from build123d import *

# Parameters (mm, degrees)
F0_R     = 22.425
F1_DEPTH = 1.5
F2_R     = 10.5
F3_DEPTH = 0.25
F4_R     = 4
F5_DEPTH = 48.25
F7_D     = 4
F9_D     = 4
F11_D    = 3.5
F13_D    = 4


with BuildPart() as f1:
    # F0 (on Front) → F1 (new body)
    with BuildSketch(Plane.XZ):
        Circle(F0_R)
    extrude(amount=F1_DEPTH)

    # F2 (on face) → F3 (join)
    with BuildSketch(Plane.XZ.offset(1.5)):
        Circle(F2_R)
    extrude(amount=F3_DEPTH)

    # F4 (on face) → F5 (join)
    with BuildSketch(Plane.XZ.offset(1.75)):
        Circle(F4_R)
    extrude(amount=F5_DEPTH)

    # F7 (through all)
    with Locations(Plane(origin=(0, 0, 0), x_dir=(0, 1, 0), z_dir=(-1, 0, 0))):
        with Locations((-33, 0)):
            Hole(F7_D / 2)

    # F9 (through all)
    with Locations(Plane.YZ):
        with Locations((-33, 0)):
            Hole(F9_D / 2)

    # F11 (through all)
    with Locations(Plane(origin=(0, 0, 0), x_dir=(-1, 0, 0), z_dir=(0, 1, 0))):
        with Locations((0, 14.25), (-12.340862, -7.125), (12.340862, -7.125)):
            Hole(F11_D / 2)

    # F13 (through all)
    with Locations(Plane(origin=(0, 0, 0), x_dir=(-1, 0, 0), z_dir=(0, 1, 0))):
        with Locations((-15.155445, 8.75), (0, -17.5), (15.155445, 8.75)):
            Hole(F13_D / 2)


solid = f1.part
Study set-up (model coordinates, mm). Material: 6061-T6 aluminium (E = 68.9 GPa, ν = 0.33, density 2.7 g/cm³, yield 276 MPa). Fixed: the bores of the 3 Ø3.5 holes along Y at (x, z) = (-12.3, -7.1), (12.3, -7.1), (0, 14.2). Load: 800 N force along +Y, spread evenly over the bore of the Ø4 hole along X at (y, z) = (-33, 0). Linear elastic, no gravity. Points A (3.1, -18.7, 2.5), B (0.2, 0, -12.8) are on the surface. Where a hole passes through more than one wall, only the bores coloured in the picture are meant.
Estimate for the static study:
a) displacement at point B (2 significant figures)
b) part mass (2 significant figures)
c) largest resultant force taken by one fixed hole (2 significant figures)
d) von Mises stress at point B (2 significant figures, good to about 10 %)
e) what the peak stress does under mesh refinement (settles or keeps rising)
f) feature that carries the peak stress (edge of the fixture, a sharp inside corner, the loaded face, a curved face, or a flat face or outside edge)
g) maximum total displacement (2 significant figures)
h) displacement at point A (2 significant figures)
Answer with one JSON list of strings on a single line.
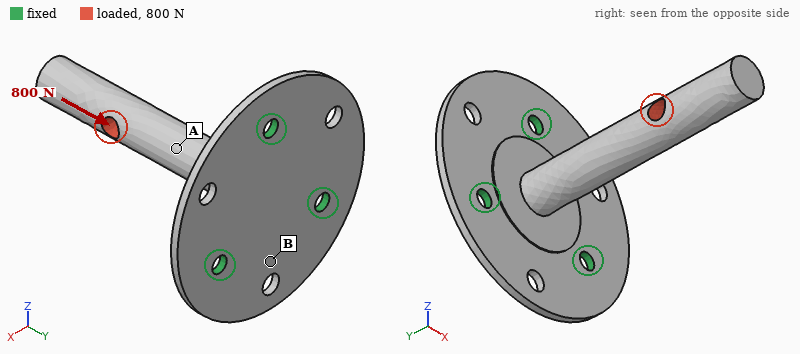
["28 µm", "13 g", "310 N", "52 MPa", "keeps rising", "edge of the fixture", "81 µm", "76 µm"]
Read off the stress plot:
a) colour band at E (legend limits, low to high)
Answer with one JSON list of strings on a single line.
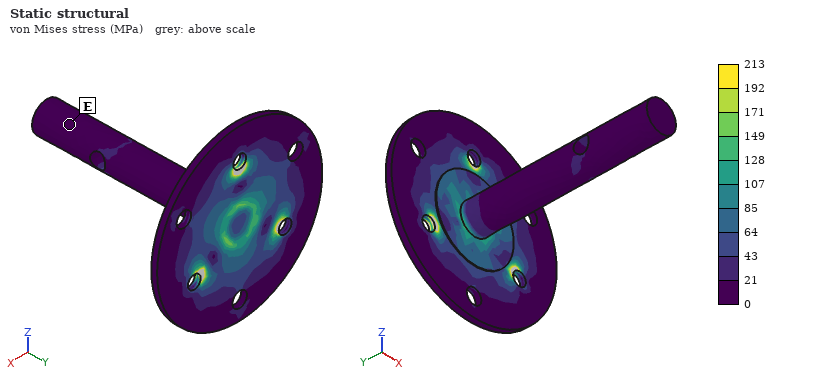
["0 to 21 MPa"]
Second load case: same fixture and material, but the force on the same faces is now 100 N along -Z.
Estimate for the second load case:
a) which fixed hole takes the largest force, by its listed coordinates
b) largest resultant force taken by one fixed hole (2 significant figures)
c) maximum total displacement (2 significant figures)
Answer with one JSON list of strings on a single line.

["(0, 14.2)", "180 N", "0.43 mm"]
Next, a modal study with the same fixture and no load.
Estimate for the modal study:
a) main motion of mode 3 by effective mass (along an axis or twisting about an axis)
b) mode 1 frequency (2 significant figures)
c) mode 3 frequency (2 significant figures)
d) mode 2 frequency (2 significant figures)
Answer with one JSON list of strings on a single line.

["along Y", "1400 Hz", "6000 Hz", "1400 Hz"]
